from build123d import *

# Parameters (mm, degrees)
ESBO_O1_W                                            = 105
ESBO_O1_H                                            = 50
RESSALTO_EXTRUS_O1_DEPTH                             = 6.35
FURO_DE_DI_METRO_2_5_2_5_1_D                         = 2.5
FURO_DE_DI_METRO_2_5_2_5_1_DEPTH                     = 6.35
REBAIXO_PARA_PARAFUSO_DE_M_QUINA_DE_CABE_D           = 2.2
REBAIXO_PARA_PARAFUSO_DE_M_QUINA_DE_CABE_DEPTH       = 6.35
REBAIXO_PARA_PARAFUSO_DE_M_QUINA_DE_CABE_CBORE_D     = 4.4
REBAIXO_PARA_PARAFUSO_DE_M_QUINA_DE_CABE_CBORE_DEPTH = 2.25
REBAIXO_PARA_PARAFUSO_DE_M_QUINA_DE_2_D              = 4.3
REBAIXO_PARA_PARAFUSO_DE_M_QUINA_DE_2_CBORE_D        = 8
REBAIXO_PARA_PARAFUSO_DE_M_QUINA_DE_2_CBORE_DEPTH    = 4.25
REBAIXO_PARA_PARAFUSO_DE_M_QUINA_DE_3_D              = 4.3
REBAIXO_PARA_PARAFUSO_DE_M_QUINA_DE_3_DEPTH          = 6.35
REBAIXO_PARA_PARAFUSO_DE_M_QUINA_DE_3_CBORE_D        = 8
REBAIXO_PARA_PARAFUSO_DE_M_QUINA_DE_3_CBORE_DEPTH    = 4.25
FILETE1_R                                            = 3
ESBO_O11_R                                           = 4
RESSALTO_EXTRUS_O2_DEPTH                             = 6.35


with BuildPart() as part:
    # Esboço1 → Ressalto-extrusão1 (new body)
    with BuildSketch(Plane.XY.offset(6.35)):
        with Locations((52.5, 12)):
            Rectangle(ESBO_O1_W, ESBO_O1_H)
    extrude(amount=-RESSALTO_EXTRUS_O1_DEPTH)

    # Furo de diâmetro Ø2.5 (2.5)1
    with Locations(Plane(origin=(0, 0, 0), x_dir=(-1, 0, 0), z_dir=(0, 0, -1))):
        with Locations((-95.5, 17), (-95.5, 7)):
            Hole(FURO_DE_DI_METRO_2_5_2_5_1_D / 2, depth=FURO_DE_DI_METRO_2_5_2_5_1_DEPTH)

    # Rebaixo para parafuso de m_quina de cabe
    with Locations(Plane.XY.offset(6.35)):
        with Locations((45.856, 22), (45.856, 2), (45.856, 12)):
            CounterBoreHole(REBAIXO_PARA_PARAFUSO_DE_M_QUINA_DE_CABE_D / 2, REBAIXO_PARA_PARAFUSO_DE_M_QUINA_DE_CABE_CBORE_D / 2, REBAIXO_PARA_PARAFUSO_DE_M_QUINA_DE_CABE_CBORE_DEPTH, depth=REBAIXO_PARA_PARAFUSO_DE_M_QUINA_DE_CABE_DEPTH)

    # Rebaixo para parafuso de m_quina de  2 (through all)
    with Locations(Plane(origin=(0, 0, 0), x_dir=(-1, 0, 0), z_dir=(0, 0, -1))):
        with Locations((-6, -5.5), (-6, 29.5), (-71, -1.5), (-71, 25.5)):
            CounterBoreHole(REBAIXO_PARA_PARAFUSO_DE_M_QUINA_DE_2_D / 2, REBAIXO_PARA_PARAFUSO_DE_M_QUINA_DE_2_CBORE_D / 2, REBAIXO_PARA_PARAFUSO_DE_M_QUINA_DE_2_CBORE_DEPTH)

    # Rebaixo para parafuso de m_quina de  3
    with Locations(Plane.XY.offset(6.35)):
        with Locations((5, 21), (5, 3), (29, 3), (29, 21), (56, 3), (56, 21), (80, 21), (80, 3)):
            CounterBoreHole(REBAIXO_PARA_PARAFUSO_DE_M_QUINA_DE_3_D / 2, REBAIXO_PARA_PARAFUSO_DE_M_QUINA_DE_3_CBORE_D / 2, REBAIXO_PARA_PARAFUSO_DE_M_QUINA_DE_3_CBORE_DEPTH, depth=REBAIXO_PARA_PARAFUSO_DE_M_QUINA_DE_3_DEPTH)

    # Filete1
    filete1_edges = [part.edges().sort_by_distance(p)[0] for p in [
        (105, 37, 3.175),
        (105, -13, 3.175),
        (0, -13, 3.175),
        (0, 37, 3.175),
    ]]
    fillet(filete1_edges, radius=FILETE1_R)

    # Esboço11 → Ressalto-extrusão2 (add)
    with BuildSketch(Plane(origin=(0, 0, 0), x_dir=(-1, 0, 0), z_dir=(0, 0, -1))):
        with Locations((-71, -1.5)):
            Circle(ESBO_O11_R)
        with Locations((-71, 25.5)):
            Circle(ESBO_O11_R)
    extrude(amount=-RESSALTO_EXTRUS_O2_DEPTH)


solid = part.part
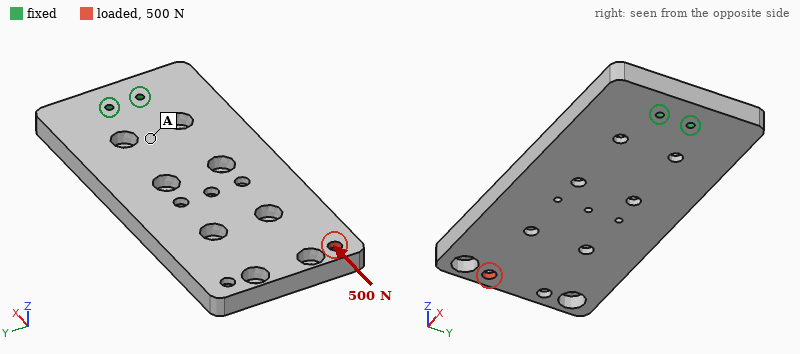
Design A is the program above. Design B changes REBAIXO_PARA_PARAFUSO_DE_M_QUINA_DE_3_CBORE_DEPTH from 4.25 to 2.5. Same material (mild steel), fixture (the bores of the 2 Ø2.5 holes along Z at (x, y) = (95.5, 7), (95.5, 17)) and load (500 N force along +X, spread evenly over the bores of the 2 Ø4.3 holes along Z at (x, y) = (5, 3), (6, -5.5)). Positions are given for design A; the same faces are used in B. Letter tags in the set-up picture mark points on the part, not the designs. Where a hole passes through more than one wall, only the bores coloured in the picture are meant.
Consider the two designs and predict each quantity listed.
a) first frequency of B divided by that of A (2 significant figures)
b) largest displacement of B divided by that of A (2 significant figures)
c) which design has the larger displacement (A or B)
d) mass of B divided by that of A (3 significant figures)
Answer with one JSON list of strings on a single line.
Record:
["0.99", "0.88", "A", "1.02"]
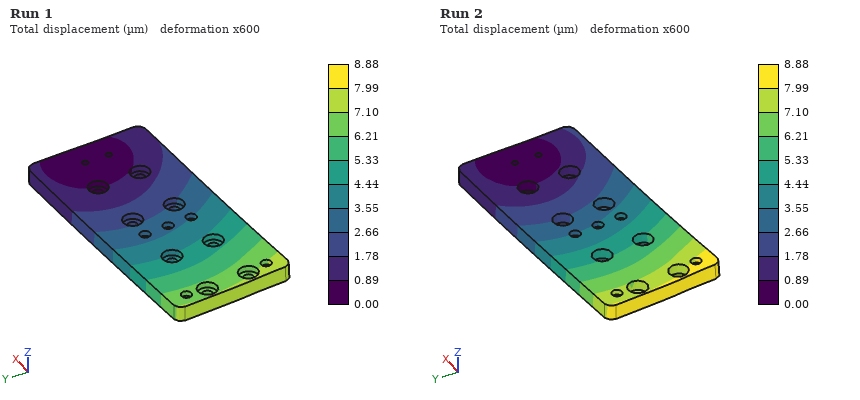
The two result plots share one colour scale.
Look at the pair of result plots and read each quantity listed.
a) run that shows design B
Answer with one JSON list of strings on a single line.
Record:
["Run 1"]
